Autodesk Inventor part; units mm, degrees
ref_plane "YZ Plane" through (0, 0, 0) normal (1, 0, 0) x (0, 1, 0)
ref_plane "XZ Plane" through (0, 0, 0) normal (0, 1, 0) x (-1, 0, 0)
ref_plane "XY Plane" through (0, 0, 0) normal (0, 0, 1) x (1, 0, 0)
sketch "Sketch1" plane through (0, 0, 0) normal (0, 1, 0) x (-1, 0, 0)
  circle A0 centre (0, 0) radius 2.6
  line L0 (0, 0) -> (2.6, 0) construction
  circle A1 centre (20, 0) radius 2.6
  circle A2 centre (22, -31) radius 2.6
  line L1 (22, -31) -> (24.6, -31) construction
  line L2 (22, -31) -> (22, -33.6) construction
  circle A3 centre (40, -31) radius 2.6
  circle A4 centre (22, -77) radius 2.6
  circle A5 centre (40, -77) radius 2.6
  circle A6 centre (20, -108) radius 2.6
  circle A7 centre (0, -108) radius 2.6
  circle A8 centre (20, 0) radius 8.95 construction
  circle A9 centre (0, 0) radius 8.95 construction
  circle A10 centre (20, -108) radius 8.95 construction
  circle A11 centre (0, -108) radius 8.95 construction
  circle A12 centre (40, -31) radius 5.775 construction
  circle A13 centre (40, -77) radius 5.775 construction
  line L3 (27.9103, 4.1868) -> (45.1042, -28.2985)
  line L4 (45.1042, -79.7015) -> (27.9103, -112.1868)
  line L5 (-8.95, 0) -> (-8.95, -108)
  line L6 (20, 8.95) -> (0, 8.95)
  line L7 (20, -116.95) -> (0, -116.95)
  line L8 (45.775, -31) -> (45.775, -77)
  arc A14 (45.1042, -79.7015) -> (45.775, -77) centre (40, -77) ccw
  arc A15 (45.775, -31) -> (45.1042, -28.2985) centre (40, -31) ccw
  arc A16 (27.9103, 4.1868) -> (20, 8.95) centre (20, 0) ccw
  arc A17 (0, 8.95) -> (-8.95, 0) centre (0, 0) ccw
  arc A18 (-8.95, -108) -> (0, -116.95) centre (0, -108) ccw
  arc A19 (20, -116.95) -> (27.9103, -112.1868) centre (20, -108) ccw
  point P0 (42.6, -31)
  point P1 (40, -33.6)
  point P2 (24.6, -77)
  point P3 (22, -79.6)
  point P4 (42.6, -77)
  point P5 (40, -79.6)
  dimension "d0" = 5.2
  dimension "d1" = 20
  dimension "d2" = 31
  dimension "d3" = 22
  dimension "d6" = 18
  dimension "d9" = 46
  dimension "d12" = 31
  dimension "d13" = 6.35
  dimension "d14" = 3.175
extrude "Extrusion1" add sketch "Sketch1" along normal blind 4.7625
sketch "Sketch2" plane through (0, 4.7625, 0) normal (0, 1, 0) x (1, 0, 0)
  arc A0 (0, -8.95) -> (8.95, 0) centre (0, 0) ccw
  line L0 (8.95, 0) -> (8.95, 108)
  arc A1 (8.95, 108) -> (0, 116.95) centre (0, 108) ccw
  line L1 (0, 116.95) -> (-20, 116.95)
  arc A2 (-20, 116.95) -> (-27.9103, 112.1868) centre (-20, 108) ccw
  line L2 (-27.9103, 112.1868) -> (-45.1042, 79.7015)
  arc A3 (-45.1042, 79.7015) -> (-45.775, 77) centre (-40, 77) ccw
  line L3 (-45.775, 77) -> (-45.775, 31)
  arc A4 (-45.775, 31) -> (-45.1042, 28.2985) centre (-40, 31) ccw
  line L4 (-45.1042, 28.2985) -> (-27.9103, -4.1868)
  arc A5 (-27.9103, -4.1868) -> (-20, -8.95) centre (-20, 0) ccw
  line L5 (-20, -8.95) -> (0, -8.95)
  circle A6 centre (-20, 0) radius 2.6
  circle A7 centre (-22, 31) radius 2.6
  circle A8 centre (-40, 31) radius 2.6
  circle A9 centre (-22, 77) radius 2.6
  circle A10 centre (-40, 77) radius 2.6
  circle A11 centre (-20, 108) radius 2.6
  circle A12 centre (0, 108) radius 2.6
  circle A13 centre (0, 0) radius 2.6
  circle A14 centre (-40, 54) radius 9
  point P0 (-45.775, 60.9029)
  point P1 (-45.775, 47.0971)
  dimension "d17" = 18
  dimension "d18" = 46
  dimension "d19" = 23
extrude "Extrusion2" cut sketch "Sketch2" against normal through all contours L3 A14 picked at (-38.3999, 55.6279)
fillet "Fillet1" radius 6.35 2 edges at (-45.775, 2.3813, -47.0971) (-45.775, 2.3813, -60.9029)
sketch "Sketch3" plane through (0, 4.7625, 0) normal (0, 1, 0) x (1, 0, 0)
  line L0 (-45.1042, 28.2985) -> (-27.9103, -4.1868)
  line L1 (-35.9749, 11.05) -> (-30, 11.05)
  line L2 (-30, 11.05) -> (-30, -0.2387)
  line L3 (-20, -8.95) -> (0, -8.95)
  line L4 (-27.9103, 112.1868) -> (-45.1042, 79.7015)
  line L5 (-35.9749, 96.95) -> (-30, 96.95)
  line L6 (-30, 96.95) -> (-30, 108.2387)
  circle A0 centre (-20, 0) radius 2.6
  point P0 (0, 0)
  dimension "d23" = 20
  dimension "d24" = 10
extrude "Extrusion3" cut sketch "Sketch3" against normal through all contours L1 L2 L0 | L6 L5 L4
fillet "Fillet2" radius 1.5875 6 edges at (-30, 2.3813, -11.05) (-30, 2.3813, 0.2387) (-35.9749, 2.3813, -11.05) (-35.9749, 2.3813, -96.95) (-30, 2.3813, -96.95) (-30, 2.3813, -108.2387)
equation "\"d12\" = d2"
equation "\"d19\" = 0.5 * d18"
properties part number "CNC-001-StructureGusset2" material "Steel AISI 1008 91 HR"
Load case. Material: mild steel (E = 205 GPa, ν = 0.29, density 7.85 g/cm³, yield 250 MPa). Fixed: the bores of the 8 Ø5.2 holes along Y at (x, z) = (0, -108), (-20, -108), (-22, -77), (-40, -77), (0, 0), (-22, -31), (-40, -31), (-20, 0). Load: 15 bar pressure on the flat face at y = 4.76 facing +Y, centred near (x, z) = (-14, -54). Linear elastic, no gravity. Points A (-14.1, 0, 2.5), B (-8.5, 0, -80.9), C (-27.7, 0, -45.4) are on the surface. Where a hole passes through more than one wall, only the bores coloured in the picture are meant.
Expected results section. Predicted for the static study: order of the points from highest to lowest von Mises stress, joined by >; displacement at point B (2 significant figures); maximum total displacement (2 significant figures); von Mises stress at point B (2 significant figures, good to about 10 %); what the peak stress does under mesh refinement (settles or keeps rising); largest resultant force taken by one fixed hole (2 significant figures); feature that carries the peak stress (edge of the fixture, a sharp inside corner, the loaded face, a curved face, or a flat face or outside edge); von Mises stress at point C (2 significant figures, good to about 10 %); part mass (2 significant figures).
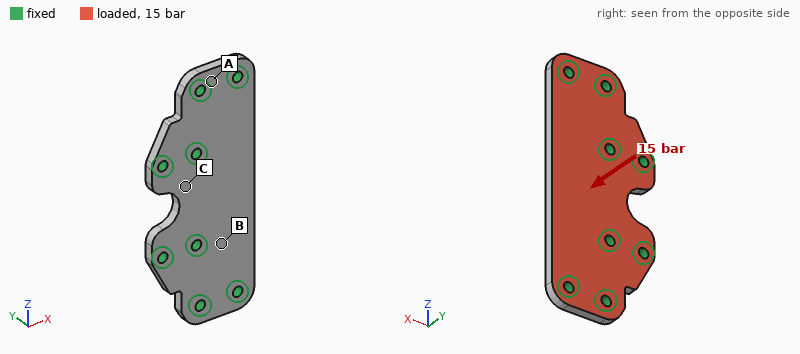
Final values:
B > C > A
17 µm
83 µm
58 MPa
keeps rising
2.3 kN
edge of the fixture
41 MPa
210 g
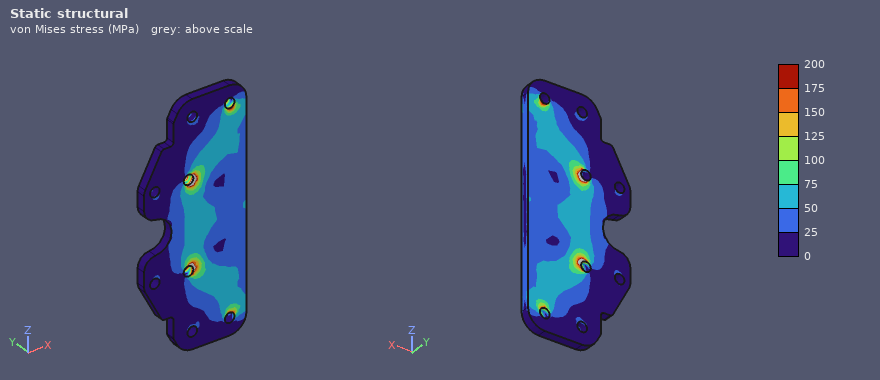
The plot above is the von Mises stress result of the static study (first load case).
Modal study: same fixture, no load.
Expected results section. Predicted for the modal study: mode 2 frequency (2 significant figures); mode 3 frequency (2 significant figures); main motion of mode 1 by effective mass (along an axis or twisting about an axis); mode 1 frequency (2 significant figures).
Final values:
8800 Hz
12 kHz
along Y
4800 Hz
